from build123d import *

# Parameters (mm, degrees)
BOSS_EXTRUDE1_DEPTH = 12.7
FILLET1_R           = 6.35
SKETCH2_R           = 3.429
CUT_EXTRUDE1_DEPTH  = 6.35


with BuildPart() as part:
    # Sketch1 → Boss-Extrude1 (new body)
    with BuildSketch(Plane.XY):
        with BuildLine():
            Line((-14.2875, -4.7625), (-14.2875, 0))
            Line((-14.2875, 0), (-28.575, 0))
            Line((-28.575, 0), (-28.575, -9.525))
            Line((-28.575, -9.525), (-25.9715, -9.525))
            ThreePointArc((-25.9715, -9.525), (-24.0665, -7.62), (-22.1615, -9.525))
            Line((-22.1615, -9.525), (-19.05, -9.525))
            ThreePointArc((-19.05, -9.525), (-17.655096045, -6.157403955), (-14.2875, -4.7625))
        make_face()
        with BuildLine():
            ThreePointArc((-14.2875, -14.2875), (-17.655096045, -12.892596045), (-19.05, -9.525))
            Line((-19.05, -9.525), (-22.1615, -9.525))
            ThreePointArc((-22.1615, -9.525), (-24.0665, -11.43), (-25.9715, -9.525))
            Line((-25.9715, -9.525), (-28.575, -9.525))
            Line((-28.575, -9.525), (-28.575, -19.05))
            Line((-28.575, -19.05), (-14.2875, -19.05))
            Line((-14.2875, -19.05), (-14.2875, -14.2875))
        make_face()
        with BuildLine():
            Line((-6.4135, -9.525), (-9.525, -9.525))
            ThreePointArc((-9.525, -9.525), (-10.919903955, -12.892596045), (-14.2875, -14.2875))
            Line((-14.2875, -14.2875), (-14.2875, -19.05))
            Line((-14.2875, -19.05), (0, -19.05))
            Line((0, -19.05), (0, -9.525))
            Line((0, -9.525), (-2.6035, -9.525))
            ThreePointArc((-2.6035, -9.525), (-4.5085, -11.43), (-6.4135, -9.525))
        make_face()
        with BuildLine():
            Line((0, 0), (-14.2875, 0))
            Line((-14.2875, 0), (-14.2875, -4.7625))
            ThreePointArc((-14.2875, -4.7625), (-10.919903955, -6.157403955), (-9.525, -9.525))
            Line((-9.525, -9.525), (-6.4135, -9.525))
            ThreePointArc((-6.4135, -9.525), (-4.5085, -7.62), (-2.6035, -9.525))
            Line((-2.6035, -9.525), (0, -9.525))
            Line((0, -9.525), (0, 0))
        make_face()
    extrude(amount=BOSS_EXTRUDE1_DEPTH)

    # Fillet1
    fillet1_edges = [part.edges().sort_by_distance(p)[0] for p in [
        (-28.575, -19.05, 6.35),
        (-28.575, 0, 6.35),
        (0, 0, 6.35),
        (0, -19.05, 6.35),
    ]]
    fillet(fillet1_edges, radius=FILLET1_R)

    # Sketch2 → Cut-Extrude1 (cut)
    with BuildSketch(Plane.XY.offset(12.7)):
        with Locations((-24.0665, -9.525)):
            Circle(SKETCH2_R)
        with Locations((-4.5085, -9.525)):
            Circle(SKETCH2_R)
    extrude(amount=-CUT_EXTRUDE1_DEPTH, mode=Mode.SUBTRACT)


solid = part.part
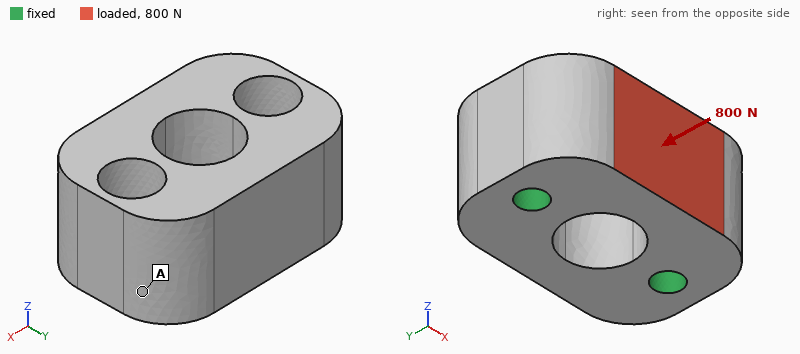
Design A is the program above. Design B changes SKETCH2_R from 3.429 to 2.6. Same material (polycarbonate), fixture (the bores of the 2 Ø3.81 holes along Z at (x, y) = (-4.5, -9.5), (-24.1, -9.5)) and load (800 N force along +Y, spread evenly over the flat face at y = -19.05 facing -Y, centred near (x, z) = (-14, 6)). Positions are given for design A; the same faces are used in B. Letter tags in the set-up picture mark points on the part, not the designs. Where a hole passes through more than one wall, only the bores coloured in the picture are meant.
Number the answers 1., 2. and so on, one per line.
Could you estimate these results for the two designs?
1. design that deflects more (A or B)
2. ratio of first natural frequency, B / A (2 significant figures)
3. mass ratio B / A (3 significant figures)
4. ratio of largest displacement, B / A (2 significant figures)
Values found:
1. A
2. 1.0
3. 1.04
4. 0.86
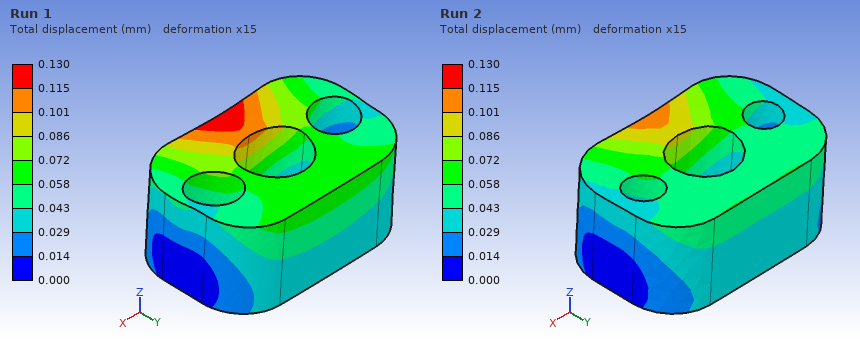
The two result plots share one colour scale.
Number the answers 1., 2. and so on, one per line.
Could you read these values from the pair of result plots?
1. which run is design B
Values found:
1. Run 2
